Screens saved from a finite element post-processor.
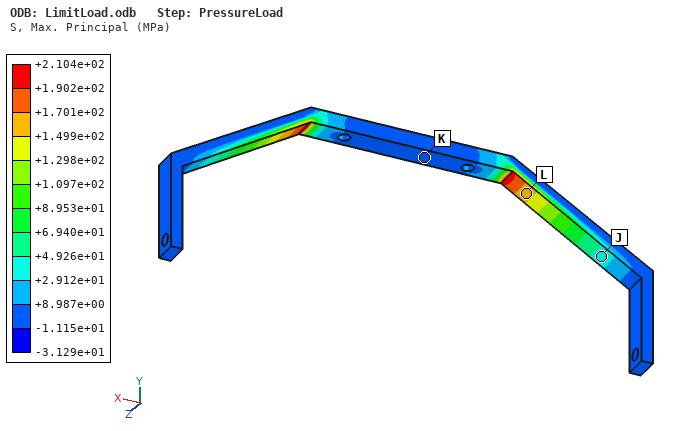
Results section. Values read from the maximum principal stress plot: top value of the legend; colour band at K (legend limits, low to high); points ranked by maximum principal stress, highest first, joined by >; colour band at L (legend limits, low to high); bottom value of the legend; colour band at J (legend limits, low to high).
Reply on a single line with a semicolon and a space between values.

+2.104e+02 MPa; -1.115e+01 to +8.987e+00 MPa; L > J > K; +1.499e+02 to +1.701e+02 MPa; -3.129e+01 MPa; +2.912e+01 to +4.926e+01 MPa
